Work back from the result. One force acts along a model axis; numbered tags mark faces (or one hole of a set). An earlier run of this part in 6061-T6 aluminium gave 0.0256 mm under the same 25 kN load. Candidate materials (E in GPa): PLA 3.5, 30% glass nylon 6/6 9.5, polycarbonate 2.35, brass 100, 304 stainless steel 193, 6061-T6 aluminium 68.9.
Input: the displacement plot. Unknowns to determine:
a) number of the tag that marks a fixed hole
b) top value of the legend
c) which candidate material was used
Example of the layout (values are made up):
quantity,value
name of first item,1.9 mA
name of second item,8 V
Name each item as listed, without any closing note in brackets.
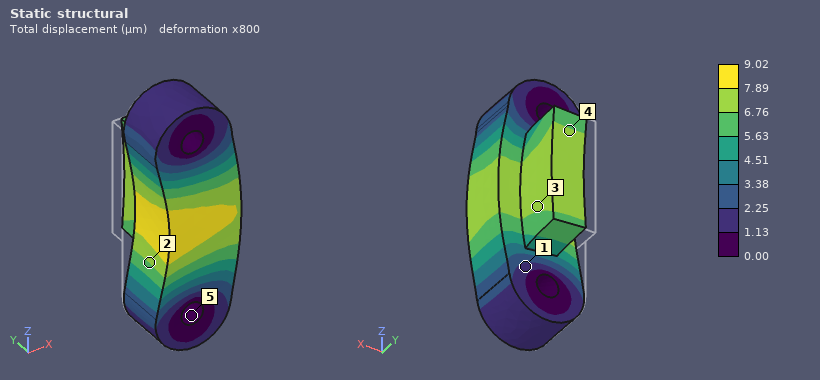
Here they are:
quantity,value
number of the tag that marks a fixed hole,5
top value of the legend,9.02 µm
which candidate material was used,304 stainless steel
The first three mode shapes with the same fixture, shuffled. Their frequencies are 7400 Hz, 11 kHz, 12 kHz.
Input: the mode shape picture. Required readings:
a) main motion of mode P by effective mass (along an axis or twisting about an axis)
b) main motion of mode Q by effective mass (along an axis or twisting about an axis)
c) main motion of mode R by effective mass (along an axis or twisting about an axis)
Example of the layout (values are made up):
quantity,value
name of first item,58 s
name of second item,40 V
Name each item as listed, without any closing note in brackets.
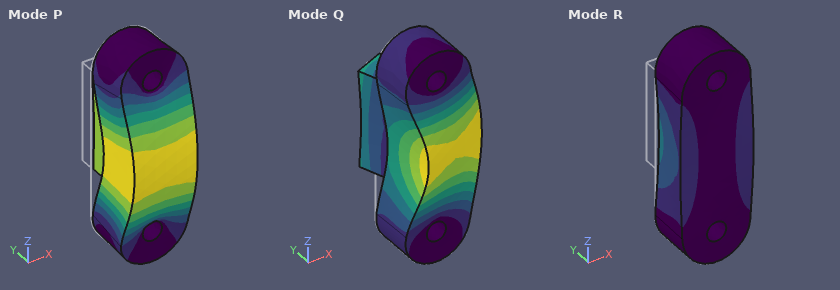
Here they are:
quantity,value
main motion of mode P by effective mass,along Y
main motion of mode Q by effective mass,along X
main motion of mode R by effective mass,along X
